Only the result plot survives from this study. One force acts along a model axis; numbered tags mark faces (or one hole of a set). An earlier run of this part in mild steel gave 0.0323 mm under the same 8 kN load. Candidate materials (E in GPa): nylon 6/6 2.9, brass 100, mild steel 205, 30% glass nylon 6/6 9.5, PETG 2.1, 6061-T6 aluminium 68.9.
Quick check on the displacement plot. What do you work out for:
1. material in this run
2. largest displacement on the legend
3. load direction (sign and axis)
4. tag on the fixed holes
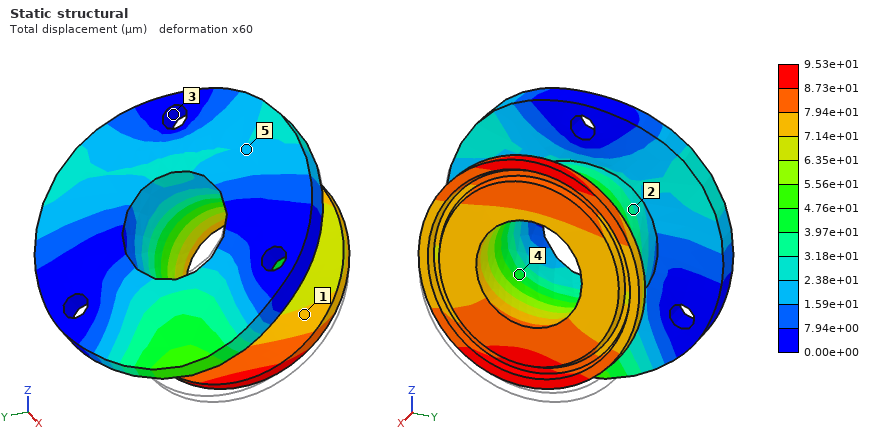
6061-T6 aluminium
9.53e+01 µm
+Z
3
